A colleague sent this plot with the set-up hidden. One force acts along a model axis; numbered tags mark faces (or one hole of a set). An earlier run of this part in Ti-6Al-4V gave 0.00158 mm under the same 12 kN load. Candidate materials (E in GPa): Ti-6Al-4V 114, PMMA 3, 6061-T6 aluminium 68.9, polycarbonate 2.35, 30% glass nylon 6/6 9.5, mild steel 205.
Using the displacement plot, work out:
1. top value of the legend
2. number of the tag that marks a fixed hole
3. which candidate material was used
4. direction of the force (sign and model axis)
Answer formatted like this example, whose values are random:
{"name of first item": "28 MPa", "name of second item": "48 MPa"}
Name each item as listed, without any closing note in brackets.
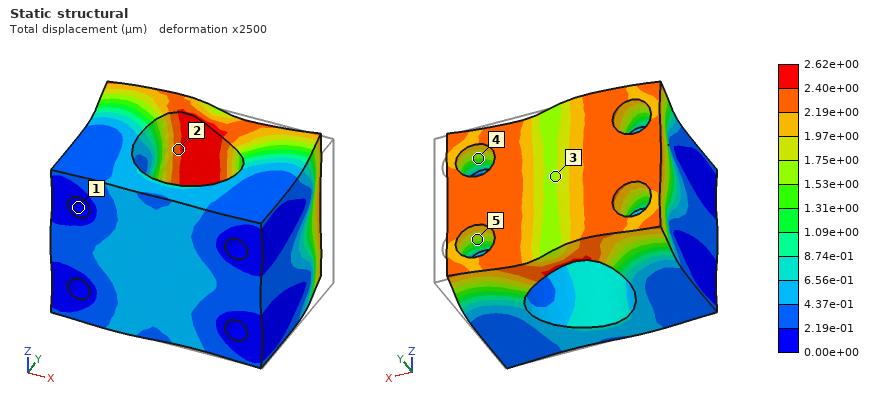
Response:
{"top value of the legend": "2.62e+00 µm", "number of the tag that marks a fixed hole": "1", "which candidate material was used": "6061-T6 aluminium", "direction of the force": "-X"}
